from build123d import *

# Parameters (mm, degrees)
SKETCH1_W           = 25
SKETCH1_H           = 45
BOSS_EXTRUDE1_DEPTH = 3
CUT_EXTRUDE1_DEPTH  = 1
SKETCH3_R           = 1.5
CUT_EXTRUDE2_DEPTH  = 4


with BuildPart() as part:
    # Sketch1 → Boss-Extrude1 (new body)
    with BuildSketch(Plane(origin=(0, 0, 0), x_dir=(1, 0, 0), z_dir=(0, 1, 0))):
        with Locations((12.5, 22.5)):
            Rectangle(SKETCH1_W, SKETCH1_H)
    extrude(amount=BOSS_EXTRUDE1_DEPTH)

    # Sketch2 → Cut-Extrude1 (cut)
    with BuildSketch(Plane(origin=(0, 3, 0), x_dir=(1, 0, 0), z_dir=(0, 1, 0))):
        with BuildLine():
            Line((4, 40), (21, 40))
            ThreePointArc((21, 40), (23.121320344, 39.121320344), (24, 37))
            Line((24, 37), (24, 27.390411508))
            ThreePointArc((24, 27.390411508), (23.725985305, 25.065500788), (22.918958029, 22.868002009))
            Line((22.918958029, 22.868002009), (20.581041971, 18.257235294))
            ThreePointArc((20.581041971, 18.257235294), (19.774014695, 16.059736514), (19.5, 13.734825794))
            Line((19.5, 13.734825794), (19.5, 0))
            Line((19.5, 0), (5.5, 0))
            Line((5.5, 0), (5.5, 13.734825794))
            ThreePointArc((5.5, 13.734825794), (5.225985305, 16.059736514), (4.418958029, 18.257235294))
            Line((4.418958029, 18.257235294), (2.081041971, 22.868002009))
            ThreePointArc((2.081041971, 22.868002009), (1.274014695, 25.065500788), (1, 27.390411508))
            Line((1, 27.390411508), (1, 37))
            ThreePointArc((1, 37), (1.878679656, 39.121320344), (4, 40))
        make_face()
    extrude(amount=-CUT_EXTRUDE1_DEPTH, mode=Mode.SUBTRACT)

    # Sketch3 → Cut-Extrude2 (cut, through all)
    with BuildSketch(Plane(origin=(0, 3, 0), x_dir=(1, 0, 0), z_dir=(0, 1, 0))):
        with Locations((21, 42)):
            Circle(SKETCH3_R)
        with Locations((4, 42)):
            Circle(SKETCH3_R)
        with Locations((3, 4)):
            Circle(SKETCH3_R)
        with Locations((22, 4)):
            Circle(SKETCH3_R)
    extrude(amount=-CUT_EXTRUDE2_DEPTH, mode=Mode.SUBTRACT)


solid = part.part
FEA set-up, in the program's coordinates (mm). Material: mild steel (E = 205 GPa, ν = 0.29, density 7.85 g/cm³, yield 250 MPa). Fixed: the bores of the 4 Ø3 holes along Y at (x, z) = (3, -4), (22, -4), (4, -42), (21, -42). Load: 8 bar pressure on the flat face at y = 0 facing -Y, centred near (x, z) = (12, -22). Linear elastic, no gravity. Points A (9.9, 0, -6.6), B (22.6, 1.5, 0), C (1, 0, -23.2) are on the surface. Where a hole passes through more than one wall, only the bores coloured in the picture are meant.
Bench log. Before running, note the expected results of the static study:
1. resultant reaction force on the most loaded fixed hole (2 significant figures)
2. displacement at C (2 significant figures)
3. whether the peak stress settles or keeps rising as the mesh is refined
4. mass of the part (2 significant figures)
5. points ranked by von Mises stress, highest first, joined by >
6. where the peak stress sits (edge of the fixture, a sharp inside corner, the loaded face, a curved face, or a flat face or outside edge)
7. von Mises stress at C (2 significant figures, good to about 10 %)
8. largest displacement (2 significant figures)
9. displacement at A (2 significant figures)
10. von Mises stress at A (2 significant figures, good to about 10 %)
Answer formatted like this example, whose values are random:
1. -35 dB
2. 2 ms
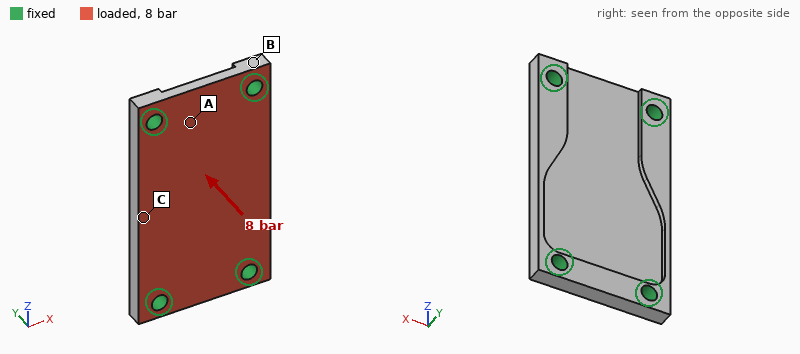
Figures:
1. 240 N
2. 17 µm
3. keeps rising
4. 20 g
5. C > A > B
6. edge of the fixture
7. 54 MPa
8. 20 µm
9. 3.2 µm
10. 30 MPa
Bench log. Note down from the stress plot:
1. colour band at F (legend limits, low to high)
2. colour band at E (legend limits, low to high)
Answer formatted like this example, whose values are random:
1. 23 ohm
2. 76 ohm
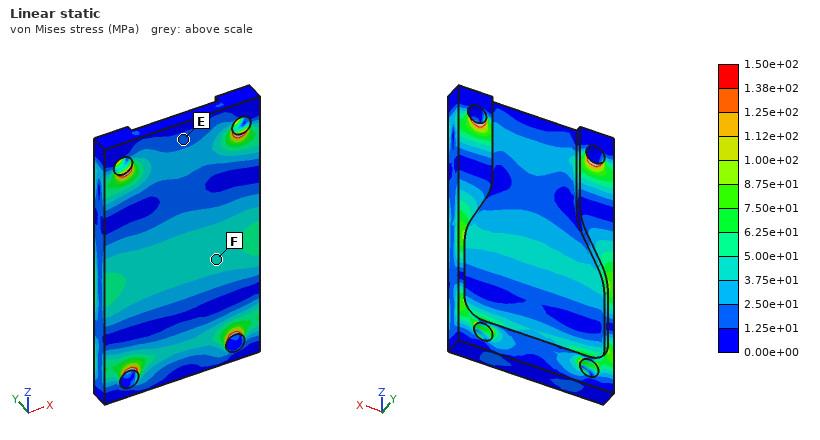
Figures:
1. 3.75e+01 to 5.00e+01 MPa
2. 1.25e+01 to 2.50e+01 MPa
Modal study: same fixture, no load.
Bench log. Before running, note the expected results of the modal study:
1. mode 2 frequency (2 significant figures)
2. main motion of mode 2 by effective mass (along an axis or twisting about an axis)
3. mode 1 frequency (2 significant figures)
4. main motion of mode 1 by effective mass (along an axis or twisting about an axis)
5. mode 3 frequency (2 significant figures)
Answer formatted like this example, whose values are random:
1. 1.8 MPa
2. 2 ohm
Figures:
1. 13 kHz
2. twisting about Z
3. 9100 Hz
4. along Y
5. 23 kHz
